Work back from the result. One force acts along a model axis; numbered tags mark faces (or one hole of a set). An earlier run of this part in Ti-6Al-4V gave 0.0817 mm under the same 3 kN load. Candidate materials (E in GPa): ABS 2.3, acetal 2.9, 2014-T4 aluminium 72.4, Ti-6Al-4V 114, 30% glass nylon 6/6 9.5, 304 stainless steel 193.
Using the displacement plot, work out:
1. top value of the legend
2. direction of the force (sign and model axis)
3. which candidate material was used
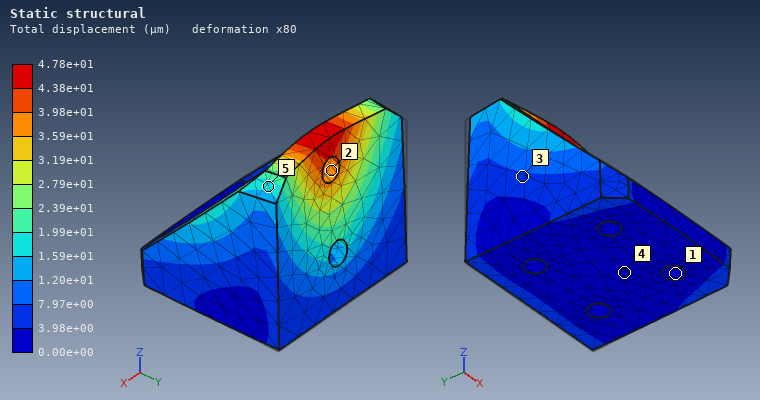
4.78e+01 µm
-Y
304 stainless steel
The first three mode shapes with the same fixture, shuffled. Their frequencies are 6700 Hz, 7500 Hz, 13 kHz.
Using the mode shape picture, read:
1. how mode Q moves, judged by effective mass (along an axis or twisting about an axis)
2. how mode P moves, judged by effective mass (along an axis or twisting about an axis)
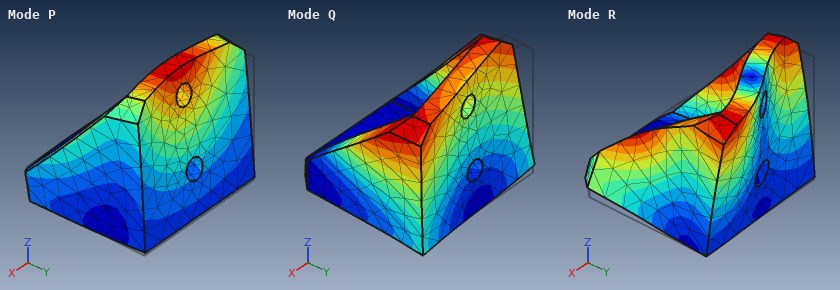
along X
along Y
